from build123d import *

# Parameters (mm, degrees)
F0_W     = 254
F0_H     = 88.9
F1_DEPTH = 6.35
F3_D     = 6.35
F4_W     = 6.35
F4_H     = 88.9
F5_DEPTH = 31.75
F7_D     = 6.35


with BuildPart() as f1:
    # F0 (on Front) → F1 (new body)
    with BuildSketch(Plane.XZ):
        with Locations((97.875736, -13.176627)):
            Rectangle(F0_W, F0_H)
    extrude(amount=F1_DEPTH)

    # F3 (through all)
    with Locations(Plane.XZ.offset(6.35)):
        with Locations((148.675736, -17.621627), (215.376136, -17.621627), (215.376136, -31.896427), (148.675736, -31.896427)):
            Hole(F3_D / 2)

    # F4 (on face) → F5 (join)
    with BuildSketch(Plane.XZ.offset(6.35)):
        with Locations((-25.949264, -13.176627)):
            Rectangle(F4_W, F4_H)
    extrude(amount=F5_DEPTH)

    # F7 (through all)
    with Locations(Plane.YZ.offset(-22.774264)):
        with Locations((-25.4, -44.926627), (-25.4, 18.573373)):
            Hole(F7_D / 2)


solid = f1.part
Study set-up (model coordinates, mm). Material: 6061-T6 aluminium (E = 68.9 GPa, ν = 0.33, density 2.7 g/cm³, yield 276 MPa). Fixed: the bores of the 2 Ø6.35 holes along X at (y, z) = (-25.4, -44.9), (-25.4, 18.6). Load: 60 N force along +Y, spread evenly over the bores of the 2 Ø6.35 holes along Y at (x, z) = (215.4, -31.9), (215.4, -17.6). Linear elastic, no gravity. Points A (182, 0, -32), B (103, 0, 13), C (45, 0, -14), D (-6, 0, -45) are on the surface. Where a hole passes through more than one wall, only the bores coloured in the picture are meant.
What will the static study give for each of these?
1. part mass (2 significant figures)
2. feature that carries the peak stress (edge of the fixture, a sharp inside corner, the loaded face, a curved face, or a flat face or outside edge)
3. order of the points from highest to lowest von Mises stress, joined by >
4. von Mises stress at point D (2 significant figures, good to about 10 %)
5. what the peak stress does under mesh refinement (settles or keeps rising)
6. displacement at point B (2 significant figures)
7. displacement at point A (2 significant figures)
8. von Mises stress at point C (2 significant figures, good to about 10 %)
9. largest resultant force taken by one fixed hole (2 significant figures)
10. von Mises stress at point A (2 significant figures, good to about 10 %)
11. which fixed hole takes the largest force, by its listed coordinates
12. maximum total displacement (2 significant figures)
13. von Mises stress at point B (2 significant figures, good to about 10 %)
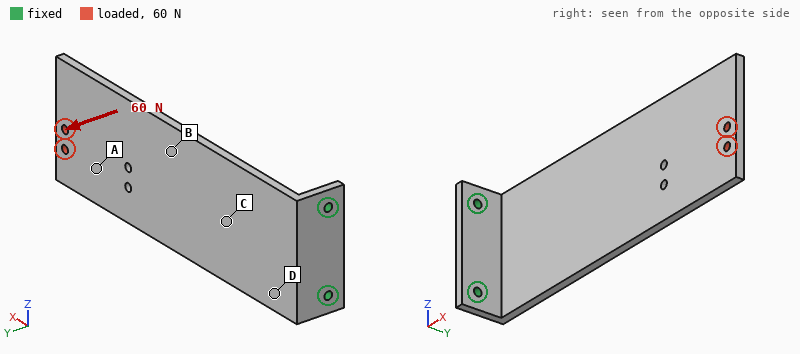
430 g
edge of the fixture
D > C > B > A
22 MPa
keeps rising
1.0 mm
2.2 mm
16 MPa
78 N
4.0 MPa
(-25.4, -44.9)
2.8 mm
11 MPa
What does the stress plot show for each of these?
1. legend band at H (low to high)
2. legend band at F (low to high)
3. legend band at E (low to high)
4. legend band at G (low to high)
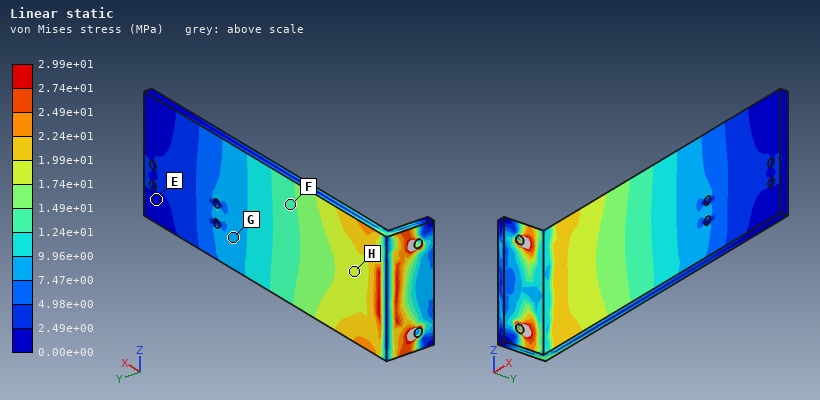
1.74e+01 to 1.99e+01 MPa
1.24e+01 to 1.49e+01 MPa
0.00e+00 to 2.49e+00 MPa
7.47e+00 to 9.96e+00 MPa
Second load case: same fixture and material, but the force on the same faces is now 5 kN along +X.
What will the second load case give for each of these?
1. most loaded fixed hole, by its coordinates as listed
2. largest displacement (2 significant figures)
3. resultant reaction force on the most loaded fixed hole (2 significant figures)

(-25.4, -44.9)
2.9 mm
3.4 kN
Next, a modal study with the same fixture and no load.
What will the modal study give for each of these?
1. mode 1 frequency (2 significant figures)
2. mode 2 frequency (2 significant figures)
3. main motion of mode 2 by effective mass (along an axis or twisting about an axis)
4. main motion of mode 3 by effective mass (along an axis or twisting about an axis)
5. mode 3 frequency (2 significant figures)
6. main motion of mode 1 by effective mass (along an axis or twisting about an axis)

73 Hz
350 Hz
along Z
along Y
460 Hz
along Y
